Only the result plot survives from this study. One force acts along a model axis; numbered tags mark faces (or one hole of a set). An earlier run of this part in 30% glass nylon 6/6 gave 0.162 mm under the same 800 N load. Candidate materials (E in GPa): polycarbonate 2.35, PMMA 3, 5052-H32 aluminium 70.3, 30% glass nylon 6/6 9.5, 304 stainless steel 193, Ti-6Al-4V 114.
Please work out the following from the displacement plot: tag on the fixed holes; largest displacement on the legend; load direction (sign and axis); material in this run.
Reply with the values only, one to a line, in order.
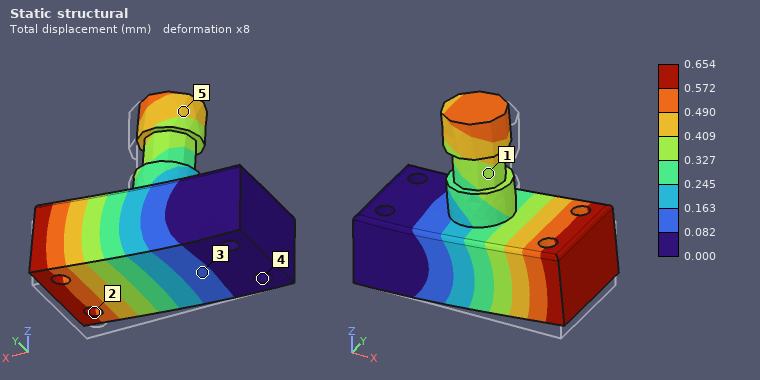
4
0.654 mm
+Z
polycarbonate
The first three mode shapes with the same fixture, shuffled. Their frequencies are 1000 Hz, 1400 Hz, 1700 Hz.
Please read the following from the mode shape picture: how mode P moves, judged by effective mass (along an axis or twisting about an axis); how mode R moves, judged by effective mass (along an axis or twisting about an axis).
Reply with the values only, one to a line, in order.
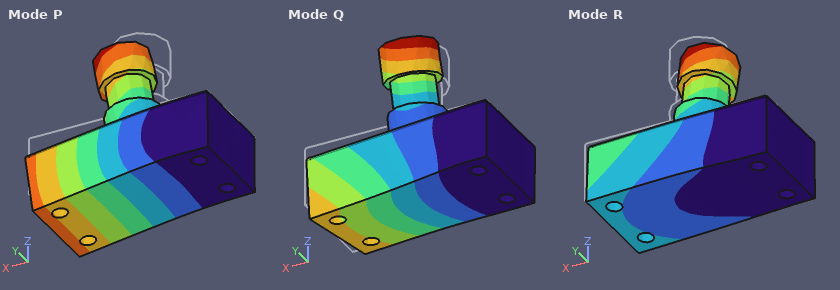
along Z
along Y
